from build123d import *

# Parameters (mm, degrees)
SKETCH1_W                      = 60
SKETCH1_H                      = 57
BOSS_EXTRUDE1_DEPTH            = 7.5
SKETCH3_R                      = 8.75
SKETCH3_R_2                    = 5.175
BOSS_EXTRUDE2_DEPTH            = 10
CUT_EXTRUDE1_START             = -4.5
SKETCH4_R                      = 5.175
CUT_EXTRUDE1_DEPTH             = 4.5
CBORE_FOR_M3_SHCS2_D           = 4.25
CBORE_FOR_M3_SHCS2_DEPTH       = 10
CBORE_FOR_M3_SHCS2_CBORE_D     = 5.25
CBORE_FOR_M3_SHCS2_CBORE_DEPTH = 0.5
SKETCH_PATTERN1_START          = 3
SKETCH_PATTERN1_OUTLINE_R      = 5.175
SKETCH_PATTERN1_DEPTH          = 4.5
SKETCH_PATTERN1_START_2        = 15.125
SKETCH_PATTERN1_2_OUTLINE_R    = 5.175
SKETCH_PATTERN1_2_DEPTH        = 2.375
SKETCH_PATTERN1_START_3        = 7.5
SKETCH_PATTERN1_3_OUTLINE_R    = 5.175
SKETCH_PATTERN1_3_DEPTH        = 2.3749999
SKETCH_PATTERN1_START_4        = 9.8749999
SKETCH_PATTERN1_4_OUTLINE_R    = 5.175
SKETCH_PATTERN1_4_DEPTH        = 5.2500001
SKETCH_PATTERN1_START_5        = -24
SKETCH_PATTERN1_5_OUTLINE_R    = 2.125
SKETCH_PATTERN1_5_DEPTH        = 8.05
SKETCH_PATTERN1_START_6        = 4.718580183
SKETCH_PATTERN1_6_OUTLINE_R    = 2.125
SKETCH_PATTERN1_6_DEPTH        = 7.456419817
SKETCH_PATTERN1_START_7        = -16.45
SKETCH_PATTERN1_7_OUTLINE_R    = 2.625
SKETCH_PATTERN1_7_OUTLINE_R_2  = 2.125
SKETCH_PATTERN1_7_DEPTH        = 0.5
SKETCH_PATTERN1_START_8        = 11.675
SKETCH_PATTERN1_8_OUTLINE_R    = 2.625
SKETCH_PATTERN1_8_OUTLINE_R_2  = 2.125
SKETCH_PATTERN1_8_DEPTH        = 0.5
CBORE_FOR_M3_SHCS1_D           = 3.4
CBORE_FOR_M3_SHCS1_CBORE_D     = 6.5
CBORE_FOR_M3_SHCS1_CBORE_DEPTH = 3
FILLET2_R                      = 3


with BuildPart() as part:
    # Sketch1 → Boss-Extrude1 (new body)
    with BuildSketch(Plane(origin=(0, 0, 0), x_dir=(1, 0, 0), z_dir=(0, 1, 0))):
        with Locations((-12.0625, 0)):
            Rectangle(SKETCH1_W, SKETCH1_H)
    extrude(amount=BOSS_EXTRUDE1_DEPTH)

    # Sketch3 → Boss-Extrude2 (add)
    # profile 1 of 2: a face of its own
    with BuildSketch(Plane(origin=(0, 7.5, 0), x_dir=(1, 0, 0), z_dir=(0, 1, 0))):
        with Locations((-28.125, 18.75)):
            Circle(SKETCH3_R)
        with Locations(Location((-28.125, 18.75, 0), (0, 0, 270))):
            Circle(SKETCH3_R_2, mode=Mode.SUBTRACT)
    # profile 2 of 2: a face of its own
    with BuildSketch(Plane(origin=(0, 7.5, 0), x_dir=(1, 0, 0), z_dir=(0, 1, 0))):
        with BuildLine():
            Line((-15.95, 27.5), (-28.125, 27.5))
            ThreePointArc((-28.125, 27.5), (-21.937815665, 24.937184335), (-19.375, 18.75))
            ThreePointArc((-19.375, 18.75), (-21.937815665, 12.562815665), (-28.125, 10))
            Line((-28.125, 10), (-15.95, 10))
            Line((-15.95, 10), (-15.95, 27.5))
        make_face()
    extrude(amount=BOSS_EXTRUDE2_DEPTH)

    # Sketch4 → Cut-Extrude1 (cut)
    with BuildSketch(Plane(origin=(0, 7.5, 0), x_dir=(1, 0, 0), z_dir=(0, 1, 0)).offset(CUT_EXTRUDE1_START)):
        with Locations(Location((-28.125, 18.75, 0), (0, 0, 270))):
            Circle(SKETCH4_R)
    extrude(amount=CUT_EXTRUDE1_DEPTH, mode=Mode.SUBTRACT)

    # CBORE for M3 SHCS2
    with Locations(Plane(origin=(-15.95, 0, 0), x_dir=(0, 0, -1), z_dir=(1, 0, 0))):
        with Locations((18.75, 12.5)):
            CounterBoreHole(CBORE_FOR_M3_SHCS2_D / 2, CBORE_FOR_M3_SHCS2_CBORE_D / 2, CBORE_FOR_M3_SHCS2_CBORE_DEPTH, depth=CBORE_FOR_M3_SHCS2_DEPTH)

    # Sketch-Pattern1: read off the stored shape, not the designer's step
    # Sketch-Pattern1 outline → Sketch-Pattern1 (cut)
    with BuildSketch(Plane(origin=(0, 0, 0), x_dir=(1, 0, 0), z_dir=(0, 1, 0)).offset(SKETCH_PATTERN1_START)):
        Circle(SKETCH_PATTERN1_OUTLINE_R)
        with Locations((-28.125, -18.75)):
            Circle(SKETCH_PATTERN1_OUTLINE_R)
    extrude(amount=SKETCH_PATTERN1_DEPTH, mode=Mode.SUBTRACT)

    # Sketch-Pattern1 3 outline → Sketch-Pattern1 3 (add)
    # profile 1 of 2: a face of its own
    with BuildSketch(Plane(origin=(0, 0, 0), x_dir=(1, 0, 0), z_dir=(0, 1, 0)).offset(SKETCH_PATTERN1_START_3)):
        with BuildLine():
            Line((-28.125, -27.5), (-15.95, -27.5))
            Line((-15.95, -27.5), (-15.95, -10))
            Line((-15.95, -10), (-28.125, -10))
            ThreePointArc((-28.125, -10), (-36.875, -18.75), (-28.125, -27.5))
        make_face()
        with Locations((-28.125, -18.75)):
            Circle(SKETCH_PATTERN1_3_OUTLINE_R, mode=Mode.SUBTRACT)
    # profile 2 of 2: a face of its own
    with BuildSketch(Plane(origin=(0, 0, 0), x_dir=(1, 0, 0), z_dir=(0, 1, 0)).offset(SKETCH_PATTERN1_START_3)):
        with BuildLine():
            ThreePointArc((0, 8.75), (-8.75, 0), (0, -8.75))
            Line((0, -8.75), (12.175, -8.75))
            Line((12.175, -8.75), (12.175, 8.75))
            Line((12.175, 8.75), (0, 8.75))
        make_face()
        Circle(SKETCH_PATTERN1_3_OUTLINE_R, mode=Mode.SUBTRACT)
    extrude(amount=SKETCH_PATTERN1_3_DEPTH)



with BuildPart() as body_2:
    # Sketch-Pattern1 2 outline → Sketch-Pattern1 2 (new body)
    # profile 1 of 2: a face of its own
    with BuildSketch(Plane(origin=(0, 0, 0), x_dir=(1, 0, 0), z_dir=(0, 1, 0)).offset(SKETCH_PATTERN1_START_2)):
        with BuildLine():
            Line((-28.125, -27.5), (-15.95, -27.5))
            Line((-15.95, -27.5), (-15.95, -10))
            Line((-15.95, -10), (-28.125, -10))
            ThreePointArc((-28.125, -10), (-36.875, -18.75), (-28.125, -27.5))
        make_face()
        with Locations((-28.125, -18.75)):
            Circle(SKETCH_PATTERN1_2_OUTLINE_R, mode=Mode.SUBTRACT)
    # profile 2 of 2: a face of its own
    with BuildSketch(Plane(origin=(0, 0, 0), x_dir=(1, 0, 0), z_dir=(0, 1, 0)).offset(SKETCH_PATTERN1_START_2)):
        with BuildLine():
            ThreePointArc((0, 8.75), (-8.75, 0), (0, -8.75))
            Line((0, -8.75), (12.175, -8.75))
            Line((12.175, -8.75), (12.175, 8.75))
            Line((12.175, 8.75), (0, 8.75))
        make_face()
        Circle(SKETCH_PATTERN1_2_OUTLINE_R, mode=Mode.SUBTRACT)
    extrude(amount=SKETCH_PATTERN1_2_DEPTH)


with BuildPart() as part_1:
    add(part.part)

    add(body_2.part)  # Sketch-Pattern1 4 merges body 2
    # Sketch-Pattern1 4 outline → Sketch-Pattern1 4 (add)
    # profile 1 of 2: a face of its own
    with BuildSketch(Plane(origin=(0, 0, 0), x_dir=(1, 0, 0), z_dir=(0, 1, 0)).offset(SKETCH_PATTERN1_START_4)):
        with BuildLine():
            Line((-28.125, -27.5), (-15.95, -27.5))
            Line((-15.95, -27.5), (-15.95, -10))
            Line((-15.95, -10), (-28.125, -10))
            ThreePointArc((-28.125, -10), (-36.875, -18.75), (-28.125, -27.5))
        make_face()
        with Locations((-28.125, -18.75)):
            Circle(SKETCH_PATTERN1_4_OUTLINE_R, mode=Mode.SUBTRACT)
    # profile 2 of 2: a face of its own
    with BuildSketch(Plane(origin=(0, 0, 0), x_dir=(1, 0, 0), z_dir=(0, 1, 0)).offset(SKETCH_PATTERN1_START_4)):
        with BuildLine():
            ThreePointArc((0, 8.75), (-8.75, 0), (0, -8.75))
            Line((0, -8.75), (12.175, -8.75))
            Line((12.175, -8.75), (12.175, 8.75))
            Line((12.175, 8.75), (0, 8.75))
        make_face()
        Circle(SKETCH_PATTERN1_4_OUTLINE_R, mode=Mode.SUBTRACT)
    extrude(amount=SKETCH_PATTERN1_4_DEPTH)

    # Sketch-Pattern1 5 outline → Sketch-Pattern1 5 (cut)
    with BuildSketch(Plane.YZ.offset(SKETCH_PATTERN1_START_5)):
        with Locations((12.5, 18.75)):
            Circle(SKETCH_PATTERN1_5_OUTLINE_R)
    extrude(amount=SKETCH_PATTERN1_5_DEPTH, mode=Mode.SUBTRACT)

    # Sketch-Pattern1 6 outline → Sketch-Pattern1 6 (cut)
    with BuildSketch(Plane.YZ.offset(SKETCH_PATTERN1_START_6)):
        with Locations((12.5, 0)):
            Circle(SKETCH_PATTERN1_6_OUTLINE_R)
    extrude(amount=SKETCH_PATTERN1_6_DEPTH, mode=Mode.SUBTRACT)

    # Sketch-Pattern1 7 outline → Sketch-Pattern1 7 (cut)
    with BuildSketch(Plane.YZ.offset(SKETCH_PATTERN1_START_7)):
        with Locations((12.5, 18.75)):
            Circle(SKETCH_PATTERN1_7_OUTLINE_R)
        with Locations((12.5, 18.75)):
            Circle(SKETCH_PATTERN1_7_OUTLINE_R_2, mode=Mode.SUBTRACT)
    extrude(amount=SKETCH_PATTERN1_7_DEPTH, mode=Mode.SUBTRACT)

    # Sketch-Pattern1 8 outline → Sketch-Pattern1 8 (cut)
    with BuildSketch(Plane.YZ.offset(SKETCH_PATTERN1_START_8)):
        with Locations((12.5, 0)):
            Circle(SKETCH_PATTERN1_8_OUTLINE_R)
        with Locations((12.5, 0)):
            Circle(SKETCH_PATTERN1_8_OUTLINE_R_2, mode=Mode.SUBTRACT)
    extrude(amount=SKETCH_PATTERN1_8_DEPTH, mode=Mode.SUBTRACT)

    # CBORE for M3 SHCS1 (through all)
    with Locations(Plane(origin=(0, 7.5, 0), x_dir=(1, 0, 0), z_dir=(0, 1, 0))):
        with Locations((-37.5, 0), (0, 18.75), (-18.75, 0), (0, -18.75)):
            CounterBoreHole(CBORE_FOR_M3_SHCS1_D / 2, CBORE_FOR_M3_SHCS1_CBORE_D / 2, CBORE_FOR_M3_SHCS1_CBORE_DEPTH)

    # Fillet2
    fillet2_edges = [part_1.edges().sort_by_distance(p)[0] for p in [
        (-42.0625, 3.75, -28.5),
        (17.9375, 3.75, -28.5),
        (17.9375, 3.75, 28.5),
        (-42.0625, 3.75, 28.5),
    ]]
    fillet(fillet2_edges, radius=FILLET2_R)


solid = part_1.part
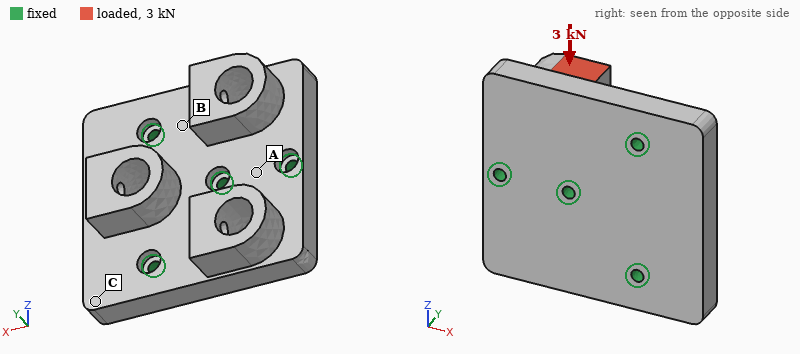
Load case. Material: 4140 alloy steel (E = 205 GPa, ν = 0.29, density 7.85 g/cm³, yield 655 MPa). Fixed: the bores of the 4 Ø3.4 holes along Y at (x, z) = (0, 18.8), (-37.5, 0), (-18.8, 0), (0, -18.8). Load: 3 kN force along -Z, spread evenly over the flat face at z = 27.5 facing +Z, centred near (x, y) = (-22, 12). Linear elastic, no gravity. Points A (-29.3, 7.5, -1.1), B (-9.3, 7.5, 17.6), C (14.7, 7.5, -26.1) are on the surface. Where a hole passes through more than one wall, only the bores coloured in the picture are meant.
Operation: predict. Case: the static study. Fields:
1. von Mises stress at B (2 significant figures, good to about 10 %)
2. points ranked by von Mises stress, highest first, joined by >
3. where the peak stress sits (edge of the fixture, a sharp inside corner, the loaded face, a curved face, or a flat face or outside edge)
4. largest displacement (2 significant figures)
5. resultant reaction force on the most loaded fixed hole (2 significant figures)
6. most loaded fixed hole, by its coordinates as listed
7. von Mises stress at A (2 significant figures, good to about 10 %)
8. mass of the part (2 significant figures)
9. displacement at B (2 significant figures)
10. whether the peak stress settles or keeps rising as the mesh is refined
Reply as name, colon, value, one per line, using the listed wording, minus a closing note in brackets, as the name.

von Mises stress at B: 56 MPa
points ranked by von Mises stress, highest first, joined by >: B > A > C
where the peak stress sits: edge of the fixture
largest displacement: 31 µm
resultant reaction force on the most loaded fixed hole: 1.5 kN
most loaded fixed hole, by its coordinates as listed: (-18.8, 0)
von Mises stress at A: 26 MPa
mass of the part: 240 g
displacement at B: 5.5 µm
whether the peak stress settles or keeps rising as the mesh is refined: keeps rising
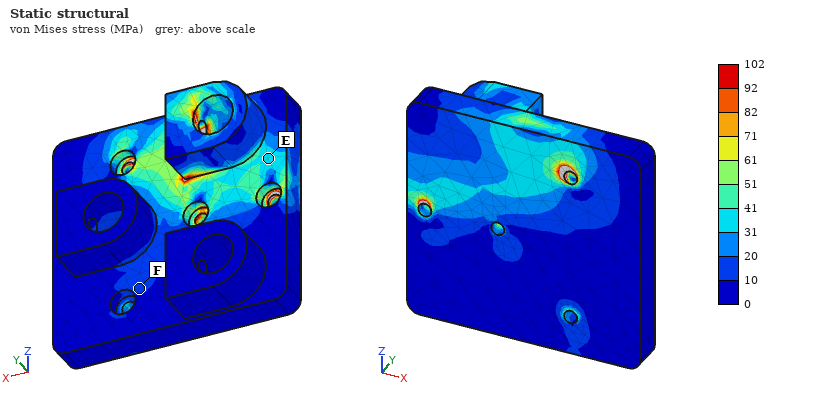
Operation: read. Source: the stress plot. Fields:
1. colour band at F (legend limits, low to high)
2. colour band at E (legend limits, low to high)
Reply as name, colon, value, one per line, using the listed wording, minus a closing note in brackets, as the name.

colour band at F: 10 to 20 MPa
colour band at E: 31 to 41 MPa
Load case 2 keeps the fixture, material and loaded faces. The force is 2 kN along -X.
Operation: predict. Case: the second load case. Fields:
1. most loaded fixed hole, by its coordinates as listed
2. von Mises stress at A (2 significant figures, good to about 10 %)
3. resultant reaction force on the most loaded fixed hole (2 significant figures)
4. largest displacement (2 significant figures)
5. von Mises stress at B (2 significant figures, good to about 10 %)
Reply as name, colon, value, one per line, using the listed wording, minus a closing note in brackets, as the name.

most loaded fixed hole, by its coordinates as listed: (0, 18.8)
von Mises stress at A: 14 MPa
resultant reaction force on the most loaded fixed hole: 1.4 kN
largest displacement: 13 µm
von Mises stress at B: 23 MPa
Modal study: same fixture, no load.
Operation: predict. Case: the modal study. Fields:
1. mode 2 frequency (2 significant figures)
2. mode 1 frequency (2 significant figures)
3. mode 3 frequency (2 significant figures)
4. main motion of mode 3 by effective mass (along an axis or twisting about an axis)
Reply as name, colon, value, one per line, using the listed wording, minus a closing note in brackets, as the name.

mode 2 frequency: 7200 Hz
mode 1 frequency: 6400 Hz
mode 3 frequency: 10 kHz
main motion of mode 3 by effective mass: along Y
